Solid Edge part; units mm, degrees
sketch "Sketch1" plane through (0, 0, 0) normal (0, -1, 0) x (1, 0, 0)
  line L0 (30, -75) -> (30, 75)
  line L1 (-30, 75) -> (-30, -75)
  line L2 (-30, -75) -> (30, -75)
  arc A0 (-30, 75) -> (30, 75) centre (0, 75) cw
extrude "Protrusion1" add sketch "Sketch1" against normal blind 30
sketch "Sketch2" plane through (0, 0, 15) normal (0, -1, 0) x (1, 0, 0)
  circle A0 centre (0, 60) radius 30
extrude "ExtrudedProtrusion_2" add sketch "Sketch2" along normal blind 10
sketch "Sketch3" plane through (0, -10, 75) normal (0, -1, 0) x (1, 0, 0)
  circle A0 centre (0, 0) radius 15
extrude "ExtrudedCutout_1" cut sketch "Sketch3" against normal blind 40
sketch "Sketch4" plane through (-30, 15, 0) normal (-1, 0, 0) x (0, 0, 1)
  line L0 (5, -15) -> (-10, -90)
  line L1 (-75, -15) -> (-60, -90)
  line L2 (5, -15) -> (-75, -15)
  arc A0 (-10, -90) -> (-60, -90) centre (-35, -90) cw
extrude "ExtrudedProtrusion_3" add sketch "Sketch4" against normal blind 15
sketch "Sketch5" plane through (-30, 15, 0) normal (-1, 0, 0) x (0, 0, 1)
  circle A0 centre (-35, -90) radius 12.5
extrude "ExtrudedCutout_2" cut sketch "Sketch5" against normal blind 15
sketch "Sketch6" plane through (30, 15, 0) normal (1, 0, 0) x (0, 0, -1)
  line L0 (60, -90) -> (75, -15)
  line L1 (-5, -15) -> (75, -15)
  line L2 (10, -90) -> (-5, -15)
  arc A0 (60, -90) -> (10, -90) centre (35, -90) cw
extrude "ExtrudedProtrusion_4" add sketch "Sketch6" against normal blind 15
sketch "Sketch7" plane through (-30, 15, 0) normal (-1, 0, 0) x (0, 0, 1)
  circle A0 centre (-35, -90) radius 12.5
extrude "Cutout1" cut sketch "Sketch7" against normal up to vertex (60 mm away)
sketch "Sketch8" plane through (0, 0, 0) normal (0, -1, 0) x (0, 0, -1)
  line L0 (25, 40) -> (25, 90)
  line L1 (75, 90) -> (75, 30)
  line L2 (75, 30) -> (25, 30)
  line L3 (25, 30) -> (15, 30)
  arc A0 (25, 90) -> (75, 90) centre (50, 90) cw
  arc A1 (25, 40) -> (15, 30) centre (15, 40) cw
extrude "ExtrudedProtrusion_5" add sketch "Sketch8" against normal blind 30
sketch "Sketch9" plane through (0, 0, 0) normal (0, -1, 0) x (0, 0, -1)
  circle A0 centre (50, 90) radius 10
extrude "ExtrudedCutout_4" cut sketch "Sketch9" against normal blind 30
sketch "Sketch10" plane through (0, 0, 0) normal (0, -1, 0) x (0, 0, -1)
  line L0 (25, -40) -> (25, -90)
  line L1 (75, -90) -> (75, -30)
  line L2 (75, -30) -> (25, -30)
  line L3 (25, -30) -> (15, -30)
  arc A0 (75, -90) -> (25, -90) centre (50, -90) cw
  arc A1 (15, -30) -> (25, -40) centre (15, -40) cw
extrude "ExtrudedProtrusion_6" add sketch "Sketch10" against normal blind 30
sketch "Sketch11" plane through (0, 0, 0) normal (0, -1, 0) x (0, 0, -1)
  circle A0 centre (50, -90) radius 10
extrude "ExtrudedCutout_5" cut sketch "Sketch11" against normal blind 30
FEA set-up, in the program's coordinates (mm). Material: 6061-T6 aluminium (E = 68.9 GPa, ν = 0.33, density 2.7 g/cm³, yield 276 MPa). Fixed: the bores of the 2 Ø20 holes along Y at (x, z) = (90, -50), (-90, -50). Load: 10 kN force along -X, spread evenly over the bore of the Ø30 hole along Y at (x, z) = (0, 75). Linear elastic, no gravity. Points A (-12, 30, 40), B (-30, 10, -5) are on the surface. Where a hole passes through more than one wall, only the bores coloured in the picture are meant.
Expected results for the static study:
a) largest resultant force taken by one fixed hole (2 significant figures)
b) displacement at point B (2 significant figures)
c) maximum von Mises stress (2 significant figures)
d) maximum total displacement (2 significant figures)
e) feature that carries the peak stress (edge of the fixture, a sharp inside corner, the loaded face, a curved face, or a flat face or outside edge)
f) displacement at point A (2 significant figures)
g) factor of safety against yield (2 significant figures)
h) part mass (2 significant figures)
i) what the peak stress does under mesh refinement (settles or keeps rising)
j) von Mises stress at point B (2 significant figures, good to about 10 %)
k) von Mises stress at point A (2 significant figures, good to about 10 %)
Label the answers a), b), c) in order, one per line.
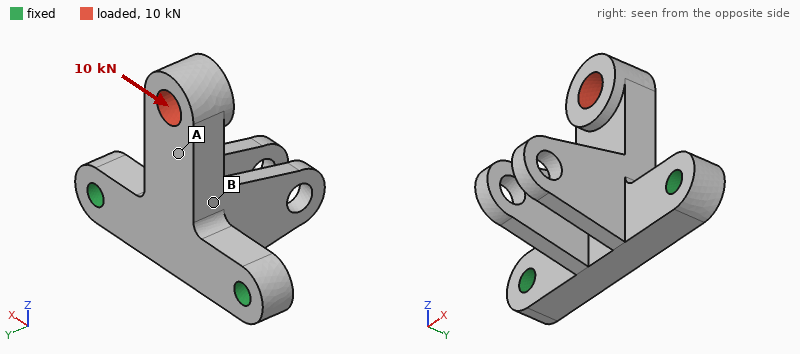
a) 9.9 kN
b) 0.046 mm
c) 88 MPa
d) 0.26 mm
e) a curved face
f) 0.10 mm
g) 3.1
h) 1.9 kg
i) settles
j) 45 MPa
k) 8.7 MPa
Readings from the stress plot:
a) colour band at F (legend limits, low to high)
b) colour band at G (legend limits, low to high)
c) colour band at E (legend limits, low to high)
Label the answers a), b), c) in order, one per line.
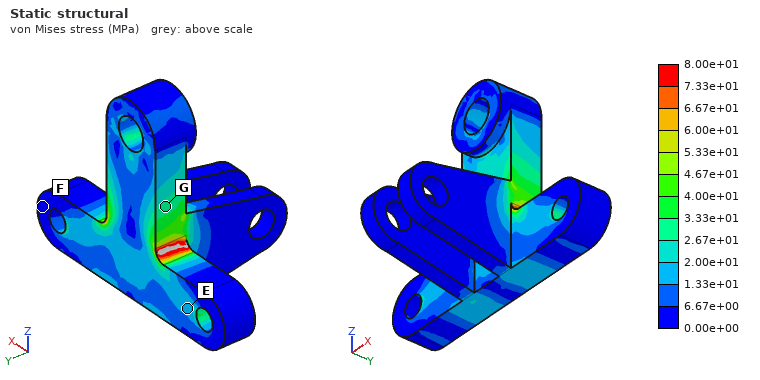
a) 0.00e+00 to 6.67e+00 MPa
b) 2.67e+01 to 3.33e+01 MPa
c) 1.33e+01 to 2.00e+01 MPa
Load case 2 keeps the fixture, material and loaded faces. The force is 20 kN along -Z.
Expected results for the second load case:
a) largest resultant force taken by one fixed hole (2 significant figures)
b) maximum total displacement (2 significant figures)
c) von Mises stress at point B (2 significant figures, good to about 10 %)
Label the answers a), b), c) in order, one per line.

a) 10 kN
b) 0.16 mm
c) 15 MPa
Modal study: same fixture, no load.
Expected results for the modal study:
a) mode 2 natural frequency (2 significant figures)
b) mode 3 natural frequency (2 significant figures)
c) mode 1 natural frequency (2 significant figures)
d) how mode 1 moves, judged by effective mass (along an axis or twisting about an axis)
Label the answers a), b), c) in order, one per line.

a) 1500 Hz
b) 1500 Hz
c) 810 Hz
d) along Y
